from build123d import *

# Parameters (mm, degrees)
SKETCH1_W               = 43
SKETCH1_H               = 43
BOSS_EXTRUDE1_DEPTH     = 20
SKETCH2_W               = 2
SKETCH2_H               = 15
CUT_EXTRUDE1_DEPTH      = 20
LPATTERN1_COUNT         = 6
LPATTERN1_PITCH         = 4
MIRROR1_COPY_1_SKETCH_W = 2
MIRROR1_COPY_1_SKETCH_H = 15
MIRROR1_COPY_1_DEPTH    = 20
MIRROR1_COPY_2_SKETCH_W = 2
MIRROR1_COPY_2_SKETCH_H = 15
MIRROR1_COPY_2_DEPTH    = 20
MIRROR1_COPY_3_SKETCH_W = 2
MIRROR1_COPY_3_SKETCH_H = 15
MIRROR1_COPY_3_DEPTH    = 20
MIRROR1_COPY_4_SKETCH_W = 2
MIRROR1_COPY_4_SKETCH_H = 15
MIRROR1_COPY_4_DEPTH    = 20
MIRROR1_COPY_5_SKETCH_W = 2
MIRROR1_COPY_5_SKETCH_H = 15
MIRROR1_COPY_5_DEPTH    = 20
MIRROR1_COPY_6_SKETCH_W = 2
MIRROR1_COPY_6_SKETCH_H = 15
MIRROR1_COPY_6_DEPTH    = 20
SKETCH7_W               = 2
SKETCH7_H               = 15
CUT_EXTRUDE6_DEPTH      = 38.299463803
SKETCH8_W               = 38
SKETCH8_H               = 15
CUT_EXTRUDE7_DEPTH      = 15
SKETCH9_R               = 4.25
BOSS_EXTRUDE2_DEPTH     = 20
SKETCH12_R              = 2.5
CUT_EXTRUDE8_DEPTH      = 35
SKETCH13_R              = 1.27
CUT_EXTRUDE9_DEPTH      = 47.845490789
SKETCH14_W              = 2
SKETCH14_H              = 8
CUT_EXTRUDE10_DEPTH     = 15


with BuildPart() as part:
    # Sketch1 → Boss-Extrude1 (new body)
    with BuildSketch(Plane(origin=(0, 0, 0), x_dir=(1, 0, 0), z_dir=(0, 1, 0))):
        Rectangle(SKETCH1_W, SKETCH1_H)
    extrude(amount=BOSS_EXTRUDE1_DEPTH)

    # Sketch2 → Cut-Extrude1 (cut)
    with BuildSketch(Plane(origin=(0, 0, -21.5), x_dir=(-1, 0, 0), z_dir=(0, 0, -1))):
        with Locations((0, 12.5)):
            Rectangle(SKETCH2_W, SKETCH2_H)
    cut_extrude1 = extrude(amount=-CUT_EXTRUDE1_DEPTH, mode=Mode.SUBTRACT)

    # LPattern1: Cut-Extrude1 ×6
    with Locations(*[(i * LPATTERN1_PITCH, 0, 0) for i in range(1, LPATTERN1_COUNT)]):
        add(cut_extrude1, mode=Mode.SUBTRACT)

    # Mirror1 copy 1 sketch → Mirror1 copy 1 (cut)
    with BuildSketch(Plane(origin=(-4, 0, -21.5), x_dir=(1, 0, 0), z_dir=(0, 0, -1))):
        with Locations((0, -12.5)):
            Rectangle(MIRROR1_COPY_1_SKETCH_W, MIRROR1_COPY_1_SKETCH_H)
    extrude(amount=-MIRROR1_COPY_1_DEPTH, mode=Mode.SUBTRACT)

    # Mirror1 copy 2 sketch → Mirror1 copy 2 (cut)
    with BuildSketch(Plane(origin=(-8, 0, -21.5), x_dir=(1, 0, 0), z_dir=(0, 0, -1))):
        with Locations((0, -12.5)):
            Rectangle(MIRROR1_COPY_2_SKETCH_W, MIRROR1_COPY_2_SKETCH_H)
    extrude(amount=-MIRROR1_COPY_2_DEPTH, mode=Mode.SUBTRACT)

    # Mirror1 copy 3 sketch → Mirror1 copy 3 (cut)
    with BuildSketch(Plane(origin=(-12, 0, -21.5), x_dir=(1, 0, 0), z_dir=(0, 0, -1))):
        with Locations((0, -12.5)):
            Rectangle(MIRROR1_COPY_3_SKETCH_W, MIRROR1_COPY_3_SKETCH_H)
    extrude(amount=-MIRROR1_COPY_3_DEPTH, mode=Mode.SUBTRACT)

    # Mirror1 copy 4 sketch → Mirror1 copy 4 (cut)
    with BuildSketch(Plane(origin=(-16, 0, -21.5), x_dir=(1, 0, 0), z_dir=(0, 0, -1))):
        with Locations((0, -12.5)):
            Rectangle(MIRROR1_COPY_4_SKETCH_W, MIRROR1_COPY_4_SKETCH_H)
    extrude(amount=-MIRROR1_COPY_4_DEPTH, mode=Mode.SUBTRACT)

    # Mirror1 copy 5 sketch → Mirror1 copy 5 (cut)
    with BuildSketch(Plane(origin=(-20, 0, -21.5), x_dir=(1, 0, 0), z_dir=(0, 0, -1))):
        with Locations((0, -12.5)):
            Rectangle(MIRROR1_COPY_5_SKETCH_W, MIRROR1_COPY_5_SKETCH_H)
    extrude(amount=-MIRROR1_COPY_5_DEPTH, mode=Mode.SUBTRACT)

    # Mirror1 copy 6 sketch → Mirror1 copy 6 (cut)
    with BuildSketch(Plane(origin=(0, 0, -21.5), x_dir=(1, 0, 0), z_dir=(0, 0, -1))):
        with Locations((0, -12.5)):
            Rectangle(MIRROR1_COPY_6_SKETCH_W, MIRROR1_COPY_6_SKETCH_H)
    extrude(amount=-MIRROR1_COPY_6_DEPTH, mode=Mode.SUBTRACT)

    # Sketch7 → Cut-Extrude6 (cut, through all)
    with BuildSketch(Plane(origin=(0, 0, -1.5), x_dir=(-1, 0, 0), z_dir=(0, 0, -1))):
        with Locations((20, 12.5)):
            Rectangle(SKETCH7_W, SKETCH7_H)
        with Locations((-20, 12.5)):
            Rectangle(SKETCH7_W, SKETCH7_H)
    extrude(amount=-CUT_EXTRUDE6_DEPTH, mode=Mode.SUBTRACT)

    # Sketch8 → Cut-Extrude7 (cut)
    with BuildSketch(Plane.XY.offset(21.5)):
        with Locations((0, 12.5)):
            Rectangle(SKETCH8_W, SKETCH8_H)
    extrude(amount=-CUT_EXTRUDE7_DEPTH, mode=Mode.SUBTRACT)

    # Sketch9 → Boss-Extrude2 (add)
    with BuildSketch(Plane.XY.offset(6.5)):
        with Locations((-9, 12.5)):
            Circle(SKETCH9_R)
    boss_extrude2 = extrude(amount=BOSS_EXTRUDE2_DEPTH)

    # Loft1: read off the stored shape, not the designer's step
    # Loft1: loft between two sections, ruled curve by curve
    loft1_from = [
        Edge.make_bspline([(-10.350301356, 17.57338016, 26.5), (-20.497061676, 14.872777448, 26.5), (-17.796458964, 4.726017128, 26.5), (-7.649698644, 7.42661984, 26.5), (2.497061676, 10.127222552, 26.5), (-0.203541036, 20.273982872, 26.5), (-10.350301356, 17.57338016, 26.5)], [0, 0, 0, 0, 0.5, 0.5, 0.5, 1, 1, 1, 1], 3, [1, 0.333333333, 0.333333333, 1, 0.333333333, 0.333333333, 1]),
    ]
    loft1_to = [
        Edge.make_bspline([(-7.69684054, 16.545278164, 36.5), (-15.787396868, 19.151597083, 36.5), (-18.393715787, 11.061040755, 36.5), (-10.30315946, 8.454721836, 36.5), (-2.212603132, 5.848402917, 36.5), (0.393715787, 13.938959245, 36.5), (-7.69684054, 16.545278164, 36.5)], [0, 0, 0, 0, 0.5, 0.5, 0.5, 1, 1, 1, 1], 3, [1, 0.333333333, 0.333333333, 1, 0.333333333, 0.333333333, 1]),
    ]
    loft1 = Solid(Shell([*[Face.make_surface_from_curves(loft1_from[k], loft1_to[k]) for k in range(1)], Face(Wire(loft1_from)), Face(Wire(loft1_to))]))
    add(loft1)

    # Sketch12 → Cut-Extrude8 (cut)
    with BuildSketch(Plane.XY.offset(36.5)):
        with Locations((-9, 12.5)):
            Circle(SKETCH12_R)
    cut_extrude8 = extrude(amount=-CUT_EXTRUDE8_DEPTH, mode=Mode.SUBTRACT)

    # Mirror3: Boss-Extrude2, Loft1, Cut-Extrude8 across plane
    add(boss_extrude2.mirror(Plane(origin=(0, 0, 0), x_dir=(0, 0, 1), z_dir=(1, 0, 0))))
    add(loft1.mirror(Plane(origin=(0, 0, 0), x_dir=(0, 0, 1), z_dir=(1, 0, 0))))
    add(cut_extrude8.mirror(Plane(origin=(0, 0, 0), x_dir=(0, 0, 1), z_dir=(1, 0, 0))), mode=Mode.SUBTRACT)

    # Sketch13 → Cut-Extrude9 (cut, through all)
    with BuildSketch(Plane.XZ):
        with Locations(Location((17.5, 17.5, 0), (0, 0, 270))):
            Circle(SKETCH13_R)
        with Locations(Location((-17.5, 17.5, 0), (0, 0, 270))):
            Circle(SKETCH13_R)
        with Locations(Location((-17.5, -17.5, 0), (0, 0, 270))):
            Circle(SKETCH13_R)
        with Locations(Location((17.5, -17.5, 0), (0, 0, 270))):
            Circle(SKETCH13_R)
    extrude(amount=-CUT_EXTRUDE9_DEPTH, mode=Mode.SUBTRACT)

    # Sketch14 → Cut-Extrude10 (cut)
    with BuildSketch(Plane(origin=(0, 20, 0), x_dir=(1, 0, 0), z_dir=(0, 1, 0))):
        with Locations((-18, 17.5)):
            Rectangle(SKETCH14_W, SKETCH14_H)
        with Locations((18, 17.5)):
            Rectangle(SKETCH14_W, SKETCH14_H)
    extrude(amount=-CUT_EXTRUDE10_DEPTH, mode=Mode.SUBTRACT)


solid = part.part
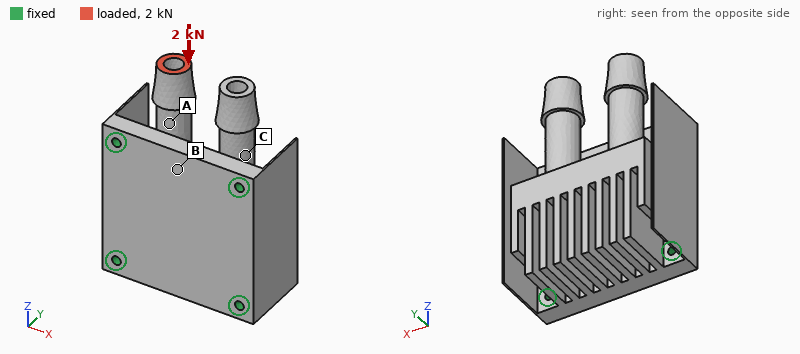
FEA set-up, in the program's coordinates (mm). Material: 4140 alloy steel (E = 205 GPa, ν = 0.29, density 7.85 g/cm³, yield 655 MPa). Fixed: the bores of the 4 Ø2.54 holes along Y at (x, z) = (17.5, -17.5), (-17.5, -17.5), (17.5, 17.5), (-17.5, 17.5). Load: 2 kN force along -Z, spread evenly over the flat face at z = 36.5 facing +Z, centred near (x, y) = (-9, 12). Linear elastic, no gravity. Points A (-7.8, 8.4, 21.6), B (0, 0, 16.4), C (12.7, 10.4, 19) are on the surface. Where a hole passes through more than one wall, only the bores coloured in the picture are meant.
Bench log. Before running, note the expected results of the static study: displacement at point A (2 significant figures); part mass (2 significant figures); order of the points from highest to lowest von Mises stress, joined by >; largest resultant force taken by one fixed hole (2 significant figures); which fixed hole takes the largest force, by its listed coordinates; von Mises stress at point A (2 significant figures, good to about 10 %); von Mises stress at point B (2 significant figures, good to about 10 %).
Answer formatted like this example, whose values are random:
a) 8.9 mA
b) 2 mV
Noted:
a) 9.0 µm
b) 170 g
c) A > B > C
d) 880 N
e) (-17.5, -17.5)
f) 53 MPa
g) 9.0 MPa
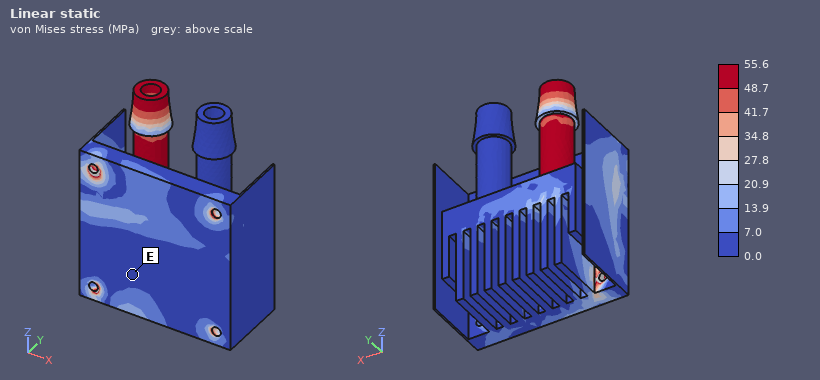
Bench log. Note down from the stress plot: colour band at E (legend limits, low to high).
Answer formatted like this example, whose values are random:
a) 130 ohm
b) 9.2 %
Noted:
a) 0.0 to 7.0 MPa
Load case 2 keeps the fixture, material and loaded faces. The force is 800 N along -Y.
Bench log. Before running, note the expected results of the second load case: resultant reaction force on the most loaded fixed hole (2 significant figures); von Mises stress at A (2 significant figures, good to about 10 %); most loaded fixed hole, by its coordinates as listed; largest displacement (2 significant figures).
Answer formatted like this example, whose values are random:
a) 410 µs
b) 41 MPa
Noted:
a) 910 N
b) 210 MPa
c) (-17.5, 17.5)
d) 0.23 mm
